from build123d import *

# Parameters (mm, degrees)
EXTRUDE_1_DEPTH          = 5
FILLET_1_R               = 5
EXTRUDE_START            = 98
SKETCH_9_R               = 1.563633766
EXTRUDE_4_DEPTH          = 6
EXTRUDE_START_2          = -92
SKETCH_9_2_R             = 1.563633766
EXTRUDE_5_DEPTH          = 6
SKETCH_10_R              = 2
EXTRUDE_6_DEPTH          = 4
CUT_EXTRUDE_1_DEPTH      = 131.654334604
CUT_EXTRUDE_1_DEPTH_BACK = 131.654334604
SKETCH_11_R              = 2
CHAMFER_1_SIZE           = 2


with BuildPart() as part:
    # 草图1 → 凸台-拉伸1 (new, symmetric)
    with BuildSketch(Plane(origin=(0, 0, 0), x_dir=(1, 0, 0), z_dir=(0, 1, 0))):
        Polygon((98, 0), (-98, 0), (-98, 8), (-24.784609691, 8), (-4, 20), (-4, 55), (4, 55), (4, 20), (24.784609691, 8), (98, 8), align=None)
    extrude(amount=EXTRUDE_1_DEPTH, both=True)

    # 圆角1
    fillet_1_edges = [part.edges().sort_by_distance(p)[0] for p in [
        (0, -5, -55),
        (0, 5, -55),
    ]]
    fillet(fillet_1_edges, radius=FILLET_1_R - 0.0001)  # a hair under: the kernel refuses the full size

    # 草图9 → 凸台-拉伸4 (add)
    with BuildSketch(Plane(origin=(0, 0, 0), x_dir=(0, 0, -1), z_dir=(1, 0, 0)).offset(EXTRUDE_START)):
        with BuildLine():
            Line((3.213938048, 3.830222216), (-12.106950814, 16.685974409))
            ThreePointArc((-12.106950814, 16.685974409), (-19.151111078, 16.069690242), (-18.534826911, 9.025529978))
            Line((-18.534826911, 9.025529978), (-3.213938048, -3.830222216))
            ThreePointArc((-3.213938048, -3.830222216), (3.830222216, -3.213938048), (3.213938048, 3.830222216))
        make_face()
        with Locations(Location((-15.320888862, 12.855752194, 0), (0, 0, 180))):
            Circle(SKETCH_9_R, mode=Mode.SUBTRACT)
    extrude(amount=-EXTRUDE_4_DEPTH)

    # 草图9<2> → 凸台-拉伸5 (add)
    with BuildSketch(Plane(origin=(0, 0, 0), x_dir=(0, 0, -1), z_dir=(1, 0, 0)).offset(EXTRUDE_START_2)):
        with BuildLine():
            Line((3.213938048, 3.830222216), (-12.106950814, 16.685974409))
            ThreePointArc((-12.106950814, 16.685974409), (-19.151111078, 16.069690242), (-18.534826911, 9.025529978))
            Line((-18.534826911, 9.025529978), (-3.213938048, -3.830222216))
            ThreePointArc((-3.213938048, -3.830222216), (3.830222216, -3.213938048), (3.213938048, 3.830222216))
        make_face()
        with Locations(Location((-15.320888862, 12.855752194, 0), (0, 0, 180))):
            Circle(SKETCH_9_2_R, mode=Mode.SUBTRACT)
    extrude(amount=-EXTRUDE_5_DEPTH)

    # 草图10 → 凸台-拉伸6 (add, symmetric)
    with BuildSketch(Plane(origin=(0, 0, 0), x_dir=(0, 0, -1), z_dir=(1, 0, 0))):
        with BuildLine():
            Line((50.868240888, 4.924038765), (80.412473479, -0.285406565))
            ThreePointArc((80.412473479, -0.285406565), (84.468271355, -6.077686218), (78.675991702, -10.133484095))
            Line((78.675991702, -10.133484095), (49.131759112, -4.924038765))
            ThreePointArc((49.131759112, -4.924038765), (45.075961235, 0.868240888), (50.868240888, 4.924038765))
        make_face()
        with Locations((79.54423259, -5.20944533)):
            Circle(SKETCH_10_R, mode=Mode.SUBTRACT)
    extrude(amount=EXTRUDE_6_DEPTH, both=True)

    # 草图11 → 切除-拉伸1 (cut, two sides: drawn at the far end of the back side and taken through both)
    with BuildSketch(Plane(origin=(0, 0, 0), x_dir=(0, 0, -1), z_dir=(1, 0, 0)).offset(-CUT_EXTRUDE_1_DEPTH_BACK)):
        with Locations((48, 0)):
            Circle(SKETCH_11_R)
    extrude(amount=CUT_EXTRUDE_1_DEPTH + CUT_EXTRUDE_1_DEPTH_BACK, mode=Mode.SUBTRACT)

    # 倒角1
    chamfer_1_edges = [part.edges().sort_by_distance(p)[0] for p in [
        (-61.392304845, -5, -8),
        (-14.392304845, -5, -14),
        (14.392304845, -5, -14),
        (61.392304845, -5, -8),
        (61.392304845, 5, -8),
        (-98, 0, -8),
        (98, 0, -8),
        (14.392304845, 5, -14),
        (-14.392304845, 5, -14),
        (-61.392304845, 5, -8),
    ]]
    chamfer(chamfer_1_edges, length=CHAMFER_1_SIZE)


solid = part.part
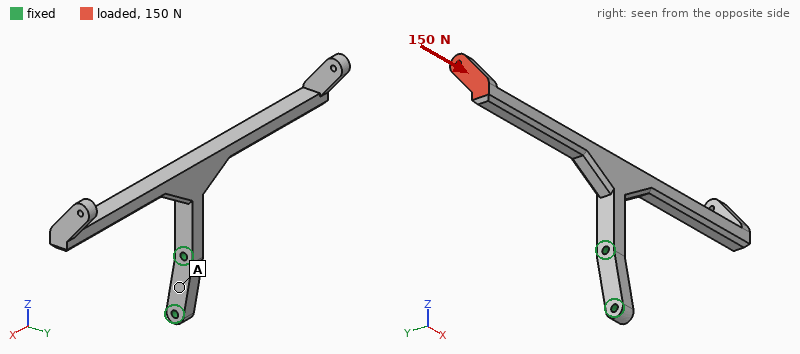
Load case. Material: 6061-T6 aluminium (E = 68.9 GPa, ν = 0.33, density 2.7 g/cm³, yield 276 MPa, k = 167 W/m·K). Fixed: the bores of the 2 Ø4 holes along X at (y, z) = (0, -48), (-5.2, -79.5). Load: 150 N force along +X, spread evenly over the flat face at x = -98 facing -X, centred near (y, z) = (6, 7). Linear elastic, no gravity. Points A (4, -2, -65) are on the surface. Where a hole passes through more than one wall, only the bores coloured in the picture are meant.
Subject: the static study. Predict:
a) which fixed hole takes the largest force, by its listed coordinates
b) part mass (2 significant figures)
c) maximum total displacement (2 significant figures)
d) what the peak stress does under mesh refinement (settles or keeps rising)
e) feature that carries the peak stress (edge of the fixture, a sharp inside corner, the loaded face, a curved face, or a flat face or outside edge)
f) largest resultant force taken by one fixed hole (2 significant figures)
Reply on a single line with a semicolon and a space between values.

(0, -48); 70 g; 0.96 mm; keeps rising; edge of the fixture; 170 N
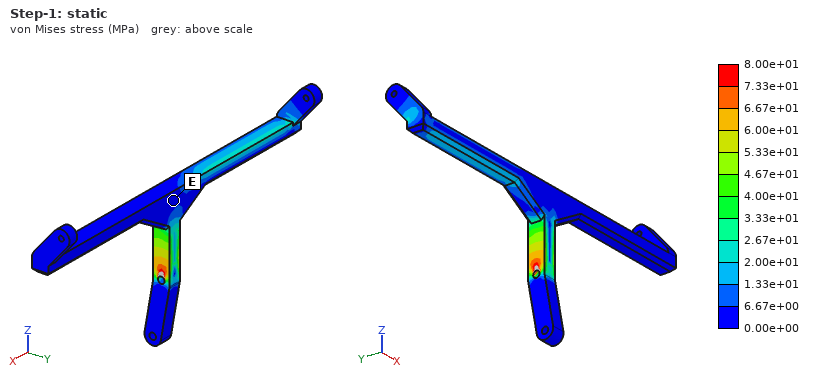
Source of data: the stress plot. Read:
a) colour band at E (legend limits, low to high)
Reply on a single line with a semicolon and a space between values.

0.00e+00 to 6.67e+00 MPa
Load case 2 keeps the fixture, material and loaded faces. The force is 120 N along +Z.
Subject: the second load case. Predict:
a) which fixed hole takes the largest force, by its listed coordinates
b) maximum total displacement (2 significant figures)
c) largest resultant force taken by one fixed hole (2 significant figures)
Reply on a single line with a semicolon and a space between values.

(0, -48); 2.3 mm; 120 N
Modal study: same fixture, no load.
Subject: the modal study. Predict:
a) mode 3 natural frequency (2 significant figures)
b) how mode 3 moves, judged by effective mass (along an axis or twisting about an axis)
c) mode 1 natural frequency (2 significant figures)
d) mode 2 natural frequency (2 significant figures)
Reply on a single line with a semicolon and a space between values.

560 Hz; along Y; 290 Hz; 290 Hz
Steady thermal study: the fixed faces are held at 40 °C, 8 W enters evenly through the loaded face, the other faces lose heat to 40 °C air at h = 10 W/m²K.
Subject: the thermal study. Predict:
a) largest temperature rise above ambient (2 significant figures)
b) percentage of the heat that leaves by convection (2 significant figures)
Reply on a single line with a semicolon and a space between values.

68 K; 28 %
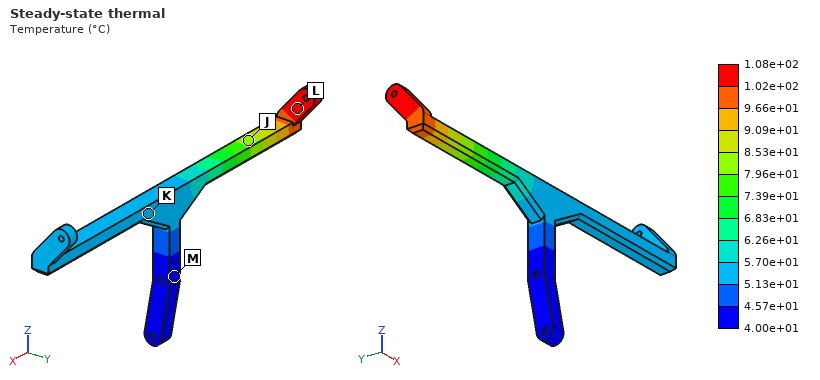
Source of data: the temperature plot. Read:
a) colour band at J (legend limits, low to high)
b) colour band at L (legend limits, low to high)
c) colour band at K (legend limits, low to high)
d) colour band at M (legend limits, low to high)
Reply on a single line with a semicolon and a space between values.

7.96e+01 to 8.53e+01 °C; 1.02e+02 to 1.08e+02 °C; 5.13e+01 to 5.70e+01 °C; 4.00e+01 to 4.57e+01 °C
